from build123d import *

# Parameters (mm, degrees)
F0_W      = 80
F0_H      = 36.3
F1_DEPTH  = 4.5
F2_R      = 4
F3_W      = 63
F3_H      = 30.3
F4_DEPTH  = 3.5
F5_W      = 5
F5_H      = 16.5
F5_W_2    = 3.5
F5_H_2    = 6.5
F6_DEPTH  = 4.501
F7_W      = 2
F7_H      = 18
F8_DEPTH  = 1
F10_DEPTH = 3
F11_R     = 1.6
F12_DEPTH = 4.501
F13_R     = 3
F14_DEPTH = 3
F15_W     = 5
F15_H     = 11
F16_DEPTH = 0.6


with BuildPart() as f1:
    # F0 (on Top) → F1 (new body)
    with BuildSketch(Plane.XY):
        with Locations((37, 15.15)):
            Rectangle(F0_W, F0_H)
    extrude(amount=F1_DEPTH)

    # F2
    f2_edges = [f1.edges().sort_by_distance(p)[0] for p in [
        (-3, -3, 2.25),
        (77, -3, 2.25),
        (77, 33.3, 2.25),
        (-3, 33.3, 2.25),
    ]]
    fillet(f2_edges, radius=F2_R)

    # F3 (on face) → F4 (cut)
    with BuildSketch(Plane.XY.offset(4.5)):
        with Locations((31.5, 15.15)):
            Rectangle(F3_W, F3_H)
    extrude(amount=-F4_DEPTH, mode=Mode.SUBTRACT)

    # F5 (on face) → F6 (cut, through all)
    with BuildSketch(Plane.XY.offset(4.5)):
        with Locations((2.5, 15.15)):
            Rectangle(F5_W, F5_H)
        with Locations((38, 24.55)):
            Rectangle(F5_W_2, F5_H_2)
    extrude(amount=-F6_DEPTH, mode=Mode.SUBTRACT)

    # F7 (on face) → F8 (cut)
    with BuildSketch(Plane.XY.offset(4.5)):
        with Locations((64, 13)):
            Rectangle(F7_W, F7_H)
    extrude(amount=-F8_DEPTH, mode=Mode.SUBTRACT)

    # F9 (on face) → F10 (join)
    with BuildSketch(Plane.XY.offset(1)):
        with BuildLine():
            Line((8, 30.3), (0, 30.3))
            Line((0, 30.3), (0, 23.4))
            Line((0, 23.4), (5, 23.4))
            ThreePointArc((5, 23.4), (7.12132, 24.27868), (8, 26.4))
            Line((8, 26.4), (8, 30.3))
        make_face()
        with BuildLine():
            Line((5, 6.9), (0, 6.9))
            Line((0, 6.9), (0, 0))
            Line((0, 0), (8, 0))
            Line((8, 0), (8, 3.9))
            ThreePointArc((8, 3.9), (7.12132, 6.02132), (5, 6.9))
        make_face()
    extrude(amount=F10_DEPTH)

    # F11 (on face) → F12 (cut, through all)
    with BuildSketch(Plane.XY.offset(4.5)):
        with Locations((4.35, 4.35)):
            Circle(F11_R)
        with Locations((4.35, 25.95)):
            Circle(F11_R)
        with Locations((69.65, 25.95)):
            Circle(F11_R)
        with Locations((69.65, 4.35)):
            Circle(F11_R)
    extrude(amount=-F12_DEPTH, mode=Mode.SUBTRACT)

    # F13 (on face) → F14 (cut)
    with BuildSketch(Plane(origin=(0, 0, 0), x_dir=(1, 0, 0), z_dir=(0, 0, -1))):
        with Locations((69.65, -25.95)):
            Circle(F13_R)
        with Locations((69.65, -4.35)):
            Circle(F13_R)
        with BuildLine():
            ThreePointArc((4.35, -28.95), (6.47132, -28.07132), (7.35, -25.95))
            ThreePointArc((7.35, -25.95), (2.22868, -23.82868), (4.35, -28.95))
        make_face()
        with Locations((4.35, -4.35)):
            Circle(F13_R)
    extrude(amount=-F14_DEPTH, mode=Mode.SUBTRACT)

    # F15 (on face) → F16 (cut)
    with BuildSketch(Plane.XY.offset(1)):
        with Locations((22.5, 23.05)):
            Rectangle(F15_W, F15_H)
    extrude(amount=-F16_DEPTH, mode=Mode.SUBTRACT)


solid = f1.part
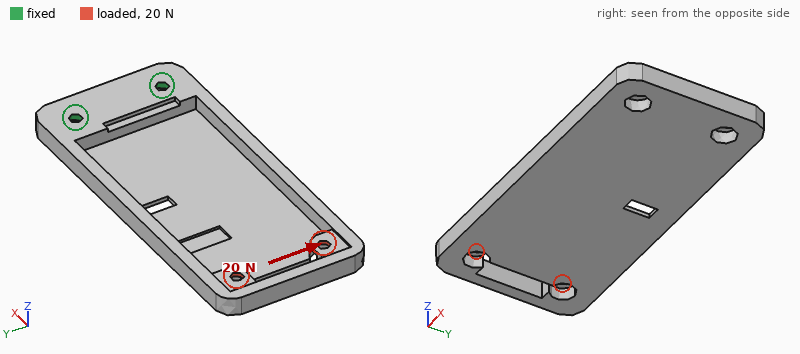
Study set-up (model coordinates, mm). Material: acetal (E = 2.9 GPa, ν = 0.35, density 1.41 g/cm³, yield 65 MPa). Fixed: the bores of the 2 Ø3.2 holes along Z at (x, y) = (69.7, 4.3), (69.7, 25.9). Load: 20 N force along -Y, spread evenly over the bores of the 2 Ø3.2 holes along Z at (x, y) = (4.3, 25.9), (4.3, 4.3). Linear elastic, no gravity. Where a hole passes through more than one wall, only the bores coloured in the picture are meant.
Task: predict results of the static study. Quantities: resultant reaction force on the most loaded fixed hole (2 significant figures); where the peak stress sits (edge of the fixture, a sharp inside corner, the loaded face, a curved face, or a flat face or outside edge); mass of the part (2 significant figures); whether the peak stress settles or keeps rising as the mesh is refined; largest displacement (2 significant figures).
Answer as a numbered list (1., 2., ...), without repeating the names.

1. 55 N
2. edge of the fixture
3. 8.6 g
4. keeps rising
5. 0.86 mm
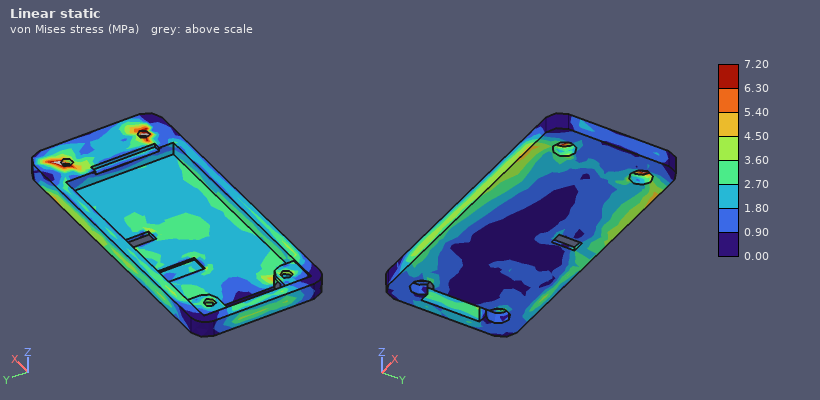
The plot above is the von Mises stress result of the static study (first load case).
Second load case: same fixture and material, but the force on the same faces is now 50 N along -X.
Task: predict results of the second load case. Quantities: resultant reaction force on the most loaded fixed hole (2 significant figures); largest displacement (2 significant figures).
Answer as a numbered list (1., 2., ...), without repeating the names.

1. 25 N
2. 1.0 mm
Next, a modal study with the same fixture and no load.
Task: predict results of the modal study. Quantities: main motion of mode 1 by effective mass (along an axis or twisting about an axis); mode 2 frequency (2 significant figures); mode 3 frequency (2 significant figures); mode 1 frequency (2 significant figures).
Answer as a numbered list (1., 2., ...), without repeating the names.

1. along Z
2. 350 Hz
3. 890 Hz
4. 150 Hz
